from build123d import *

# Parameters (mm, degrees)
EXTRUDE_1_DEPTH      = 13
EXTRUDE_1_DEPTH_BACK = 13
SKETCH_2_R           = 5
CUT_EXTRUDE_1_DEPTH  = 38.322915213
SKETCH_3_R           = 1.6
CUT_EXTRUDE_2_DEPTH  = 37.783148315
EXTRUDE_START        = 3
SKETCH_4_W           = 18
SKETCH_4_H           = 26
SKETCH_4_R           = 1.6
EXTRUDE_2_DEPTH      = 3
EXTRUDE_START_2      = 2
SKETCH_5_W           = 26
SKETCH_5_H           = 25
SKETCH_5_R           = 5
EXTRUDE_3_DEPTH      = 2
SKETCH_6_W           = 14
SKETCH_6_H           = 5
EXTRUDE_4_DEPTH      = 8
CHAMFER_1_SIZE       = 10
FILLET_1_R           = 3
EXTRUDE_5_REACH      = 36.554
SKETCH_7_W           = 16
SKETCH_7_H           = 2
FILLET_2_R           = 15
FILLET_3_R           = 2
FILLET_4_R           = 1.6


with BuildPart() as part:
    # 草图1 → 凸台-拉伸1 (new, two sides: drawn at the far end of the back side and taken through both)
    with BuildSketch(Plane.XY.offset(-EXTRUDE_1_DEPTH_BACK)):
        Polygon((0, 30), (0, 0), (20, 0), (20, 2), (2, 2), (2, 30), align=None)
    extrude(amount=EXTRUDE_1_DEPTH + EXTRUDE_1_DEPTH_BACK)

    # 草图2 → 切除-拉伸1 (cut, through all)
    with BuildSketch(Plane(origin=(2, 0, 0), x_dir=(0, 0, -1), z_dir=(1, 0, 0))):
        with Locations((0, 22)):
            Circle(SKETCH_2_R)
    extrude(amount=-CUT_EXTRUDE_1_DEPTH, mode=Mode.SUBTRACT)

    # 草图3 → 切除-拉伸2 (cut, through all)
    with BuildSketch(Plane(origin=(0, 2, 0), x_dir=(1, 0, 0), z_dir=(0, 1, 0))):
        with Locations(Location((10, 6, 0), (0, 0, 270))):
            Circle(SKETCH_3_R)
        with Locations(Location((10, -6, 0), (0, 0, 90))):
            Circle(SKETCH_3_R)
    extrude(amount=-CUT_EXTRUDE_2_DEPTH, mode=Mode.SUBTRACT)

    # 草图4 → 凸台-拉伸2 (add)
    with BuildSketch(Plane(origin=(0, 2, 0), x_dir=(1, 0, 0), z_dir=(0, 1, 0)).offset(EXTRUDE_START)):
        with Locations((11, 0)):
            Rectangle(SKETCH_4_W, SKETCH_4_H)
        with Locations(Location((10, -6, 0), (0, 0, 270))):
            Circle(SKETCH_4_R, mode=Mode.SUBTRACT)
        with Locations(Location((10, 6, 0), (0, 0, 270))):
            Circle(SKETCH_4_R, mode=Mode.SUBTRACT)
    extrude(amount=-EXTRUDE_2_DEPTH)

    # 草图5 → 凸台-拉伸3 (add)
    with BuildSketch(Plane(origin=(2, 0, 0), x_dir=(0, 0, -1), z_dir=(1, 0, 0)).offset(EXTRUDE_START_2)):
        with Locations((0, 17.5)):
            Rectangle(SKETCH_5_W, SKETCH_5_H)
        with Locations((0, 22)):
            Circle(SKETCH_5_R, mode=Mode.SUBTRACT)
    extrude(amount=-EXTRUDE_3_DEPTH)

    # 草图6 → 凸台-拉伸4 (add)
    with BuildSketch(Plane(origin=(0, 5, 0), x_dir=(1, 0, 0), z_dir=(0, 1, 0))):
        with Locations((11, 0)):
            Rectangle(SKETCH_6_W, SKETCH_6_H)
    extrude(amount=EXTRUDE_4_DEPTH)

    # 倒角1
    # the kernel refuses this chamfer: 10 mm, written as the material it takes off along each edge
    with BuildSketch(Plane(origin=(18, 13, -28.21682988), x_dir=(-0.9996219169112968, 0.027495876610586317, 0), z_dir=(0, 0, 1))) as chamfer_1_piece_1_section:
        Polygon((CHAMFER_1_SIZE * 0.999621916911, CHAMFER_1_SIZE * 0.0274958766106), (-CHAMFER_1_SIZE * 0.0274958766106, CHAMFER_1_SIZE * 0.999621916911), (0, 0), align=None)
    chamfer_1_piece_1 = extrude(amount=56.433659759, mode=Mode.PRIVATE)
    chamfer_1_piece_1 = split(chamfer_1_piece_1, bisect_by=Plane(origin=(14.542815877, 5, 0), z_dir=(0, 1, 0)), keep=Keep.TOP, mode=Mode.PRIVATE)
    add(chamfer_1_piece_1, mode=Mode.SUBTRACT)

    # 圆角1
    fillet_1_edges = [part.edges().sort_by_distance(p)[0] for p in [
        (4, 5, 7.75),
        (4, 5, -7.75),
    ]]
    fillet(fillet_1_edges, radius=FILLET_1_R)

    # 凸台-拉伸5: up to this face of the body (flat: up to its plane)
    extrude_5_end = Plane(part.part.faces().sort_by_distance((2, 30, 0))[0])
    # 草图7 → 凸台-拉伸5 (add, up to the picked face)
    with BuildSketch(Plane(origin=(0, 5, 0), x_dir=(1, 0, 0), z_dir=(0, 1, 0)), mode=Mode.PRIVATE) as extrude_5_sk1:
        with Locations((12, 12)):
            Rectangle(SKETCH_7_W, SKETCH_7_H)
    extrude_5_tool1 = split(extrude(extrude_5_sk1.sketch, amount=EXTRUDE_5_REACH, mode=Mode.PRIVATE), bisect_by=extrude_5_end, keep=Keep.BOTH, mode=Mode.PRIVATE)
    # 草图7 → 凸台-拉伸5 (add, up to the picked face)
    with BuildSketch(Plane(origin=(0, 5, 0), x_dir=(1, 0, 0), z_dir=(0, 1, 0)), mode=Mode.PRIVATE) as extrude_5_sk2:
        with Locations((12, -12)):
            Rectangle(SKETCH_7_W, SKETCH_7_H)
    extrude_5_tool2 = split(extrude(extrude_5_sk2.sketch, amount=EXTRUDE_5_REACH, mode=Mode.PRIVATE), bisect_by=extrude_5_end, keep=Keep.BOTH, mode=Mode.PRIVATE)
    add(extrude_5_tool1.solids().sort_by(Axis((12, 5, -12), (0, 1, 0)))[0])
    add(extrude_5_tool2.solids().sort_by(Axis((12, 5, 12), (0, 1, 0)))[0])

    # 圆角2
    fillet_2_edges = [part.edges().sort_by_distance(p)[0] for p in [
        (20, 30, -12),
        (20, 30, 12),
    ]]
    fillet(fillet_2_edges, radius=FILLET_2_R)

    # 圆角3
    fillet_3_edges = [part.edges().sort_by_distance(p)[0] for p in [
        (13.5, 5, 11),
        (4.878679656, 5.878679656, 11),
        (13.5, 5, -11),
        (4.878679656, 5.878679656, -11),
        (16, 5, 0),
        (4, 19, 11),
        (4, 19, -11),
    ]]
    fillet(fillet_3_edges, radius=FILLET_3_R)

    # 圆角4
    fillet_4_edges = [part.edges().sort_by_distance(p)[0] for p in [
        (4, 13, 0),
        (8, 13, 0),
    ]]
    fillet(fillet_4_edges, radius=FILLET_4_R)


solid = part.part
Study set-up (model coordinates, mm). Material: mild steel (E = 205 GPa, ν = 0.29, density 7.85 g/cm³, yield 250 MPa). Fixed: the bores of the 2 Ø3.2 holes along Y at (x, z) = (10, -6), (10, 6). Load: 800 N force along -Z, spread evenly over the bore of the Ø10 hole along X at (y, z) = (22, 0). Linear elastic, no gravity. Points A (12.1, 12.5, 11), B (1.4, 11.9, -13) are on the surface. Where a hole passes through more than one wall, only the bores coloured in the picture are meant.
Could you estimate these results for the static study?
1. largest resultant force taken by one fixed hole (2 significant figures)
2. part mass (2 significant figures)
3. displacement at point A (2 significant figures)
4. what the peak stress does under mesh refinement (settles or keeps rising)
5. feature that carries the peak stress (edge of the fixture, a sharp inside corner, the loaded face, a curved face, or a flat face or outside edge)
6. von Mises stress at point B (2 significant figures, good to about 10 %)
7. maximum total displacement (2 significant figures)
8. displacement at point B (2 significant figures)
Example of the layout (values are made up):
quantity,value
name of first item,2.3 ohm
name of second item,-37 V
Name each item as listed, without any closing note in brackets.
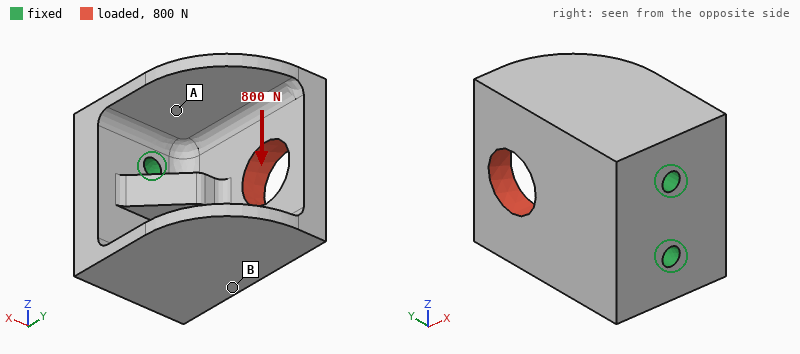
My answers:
quantity,value
largest resultant force taken by one fixed hole,1.1 kN
part mass,52 g
displacement at point A,4.9 µm
what the peak stress does under mesh refinement,keeps rising
feature that carries the peak stress,edge of the fixture
von Mises stress at point B,17 MPa
maximum total displacement,18 µm
displacement at point B,6.6 µm
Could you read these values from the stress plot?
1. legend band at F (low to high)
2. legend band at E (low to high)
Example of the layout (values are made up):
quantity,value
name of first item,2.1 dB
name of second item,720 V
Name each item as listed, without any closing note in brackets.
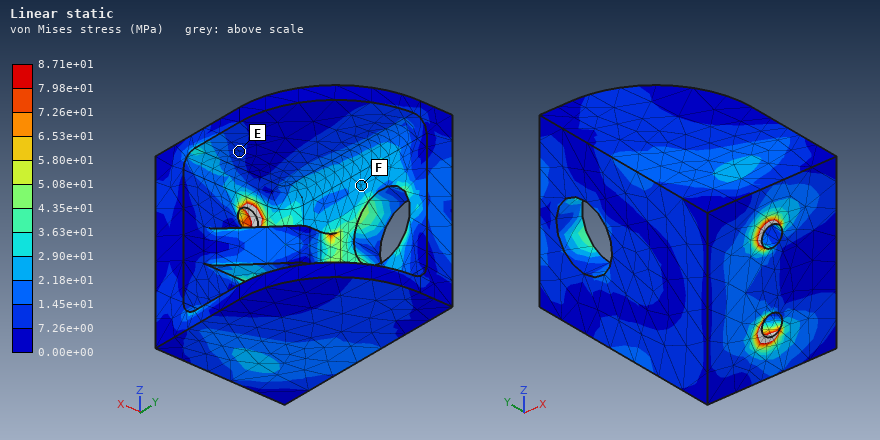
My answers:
quantity,value
legend band at F,2.18e+01 to 2.90e+01 MPa
legend band at E,7.26e+00 to 1.45e+01 MPa
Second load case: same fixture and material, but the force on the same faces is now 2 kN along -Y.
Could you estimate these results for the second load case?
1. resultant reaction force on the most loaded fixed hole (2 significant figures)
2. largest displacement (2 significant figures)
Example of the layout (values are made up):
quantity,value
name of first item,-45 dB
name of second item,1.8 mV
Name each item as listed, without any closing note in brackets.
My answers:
quantity,value
resultant reaction force on the most loaded fixed hole,1.0 kN
largest displacement,22 µm
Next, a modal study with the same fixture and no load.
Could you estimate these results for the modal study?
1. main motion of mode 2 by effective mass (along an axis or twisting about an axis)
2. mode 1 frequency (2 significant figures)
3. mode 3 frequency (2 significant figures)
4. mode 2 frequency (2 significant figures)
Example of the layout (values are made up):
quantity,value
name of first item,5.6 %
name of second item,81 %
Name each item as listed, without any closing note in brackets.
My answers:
quantity,value
main motion of mode 2 by effective mass,along Z
mode 1 frequency,7400 Hz
mode 3 frequency,11 kHz
mode 2 frequency,7700 Hz
